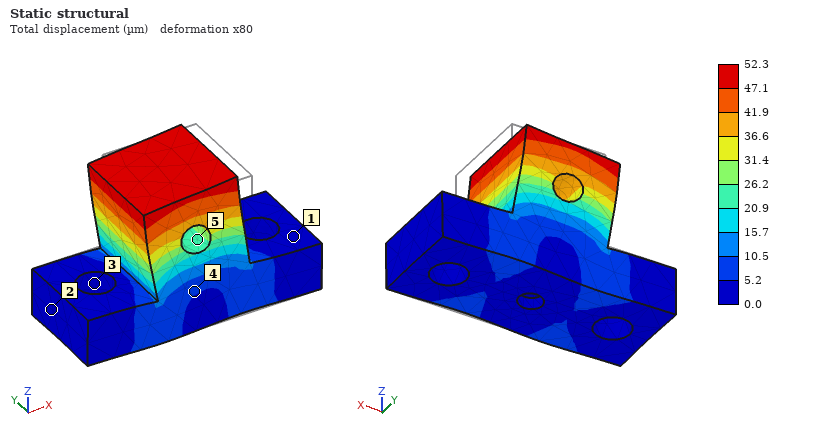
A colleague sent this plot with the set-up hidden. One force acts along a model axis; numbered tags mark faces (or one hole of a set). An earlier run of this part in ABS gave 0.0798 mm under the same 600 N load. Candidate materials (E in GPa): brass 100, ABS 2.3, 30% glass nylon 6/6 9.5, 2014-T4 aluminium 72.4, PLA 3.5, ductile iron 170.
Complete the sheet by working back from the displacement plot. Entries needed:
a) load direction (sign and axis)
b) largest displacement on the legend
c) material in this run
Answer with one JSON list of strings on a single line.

["-X", "52.3 µm", "PLA"]
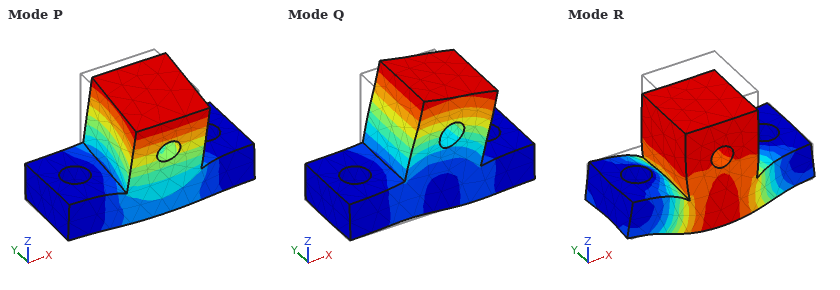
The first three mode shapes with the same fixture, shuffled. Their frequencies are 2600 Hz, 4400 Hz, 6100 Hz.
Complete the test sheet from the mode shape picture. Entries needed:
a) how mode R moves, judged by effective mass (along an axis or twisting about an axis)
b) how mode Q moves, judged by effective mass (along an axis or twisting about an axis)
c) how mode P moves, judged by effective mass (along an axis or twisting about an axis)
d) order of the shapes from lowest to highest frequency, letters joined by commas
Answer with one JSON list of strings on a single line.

["along Z", "along X", "along Y", "P, Q, R"]
